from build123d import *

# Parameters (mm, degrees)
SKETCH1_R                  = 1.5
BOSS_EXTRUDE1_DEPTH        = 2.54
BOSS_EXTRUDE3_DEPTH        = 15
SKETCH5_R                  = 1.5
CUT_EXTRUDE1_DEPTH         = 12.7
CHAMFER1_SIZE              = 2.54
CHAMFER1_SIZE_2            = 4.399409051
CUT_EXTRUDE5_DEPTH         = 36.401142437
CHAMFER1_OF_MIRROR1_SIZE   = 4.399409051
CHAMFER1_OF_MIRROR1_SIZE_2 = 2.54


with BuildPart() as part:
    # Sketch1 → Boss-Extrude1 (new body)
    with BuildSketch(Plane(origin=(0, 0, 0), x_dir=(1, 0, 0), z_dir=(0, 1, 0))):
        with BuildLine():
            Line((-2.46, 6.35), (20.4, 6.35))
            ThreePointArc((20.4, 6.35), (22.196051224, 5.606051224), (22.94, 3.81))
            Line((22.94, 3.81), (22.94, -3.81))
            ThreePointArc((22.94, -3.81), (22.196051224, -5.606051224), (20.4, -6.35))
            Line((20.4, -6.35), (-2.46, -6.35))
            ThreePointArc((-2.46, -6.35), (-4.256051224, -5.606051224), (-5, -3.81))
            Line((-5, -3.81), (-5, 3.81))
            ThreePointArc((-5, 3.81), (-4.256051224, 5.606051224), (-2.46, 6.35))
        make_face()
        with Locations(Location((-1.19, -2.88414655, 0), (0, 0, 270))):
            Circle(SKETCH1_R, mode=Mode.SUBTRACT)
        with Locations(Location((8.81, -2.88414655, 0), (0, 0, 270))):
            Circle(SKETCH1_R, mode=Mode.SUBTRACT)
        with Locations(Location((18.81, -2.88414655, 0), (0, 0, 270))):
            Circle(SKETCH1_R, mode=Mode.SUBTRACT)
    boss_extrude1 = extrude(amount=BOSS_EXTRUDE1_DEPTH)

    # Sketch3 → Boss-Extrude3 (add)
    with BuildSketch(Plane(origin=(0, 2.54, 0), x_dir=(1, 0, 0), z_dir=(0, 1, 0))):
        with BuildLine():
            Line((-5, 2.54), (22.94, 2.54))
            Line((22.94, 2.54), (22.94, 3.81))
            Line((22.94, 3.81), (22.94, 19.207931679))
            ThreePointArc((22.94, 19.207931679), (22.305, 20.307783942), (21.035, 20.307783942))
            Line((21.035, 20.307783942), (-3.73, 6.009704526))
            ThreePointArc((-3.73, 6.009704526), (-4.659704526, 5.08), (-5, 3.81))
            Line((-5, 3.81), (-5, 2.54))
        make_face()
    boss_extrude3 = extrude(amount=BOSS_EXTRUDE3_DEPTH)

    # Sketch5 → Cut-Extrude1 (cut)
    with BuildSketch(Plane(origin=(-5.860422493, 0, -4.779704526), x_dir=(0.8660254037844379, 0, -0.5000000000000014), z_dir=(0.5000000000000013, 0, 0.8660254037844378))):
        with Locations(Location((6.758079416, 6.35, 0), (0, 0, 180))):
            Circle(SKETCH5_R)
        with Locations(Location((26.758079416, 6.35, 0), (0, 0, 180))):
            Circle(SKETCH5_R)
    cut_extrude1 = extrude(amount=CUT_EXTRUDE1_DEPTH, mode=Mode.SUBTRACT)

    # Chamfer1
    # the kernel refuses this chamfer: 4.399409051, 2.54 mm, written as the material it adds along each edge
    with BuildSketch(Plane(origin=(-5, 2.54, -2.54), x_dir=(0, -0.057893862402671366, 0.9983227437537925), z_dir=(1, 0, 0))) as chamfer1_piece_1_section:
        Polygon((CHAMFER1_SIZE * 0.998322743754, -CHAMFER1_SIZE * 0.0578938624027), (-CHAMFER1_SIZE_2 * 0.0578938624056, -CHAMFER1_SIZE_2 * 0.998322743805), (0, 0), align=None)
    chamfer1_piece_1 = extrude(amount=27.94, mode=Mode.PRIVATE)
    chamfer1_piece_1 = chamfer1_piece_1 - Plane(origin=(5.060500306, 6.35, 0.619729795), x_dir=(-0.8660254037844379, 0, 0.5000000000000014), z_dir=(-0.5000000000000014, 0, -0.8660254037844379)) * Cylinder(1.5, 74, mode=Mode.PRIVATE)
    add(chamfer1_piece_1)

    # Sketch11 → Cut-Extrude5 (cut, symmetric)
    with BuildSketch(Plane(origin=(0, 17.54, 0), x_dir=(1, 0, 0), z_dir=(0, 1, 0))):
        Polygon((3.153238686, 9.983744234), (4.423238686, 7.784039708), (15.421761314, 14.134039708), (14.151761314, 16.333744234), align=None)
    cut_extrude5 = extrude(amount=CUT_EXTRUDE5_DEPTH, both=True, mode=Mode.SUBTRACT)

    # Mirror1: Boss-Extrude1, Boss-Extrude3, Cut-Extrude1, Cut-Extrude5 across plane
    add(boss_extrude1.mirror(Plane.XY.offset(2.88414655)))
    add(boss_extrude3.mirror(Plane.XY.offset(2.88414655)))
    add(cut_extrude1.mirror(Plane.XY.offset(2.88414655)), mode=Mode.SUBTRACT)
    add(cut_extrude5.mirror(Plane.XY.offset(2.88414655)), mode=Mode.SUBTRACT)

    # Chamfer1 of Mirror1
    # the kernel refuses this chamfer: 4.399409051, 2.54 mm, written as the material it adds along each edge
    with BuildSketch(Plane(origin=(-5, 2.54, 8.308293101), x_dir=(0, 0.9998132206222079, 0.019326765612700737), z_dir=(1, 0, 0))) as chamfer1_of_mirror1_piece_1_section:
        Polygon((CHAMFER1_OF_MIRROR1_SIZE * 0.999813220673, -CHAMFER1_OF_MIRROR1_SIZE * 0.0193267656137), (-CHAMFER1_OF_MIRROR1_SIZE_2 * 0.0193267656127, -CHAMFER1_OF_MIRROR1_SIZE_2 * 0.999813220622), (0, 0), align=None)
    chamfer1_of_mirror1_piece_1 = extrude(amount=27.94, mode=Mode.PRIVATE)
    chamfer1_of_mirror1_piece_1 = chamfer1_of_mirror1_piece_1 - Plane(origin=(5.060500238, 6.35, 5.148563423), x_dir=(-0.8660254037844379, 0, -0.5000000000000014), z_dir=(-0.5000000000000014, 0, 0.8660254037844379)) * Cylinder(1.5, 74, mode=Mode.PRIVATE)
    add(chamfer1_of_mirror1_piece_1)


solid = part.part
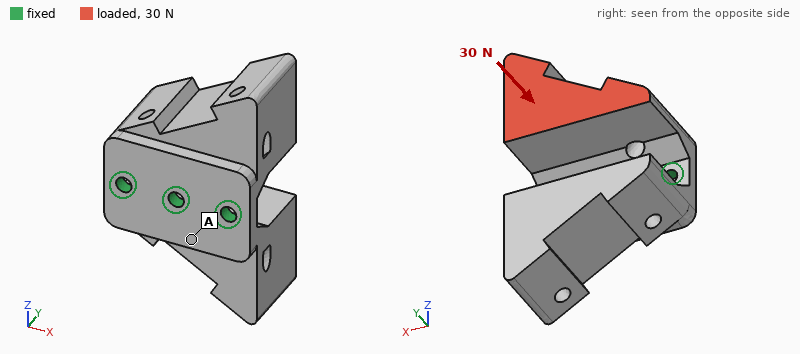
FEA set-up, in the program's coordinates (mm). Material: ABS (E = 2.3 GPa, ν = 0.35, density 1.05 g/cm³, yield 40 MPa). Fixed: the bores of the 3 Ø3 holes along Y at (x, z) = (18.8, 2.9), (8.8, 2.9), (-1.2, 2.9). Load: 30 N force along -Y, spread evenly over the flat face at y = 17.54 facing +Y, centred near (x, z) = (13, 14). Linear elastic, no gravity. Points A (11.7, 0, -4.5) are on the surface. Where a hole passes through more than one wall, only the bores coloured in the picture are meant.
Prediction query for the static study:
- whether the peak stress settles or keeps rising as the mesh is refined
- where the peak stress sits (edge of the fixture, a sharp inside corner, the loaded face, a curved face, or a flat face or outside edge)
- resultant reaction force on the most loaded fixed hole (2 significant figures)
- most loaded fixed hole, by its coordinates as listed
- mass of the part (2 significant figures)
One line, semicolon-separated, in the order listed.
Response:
keeps rising; edge of the fixture; 16 N; (18.8, 2.9); 9.8 g
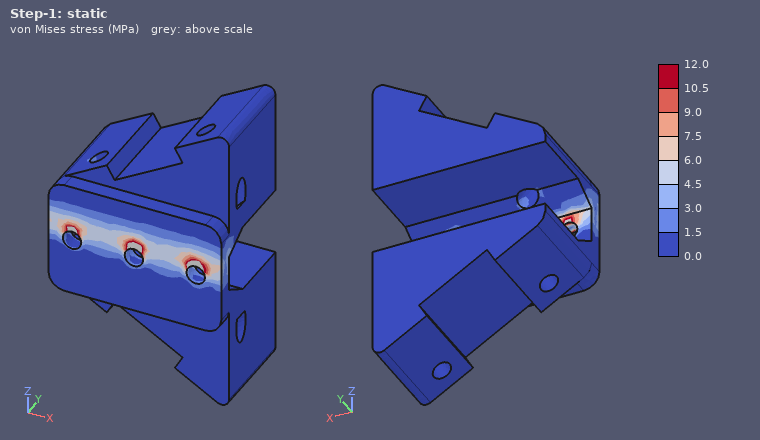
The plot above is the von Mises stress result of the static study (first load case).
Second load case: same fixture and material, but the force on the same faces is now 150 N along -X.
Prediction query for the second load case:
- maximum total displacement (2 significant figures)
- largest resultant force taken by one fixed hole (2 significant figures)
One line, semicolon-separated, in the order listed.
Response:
0.21 mm; 150 N
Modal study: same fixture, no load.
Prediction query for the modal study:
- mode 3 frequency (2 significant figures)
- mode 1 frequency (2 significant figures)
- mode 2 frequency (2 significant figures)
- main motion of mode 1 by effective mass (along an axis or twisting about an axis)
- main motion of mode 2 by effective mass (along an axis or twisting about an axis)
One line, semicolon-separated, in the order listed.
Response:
3200 Hz; 840 Hz; 880 Hz; along Z; along Y
